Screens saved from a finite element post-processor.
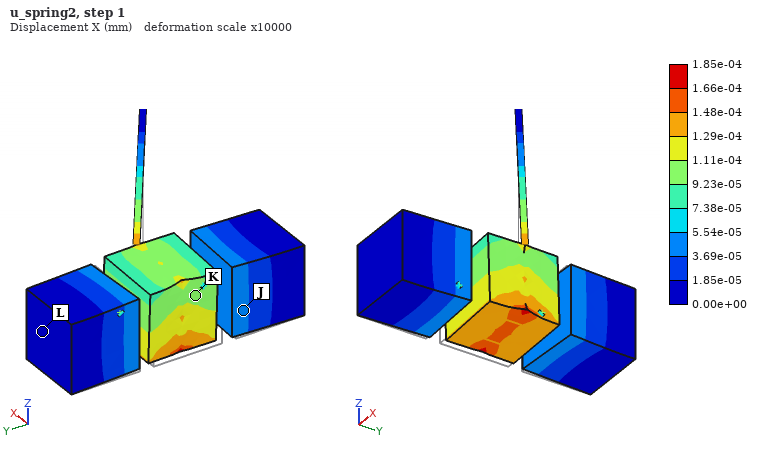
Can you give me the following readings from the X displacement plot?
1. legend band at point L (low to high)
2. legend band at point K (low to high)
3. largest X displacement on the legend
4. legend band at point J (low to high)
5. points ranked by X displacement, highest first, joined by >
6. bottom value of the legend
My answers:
0.00e+00 to 1.85e-05 mm
9.23e-05 to 1.11e-04 mm
1.85e-04 mm
3.69e-05 to 5.54e-05 mm
K > J > L
0.00e+00 mm
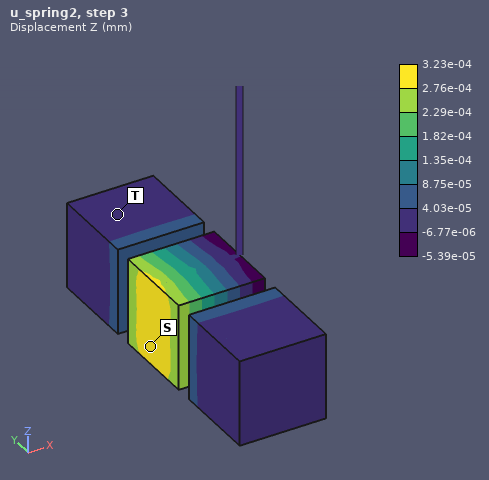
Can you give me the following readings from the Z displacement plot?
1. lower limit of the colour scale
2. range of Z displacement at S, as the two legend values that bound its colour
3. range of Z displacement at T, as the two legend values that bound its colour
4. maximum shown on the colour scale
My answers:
-5.39e-05 mm
2.76e-04 to 3.23e-04 mm
-6.77e-06 to 4.03e-05 mm
3.23e-04 mm
